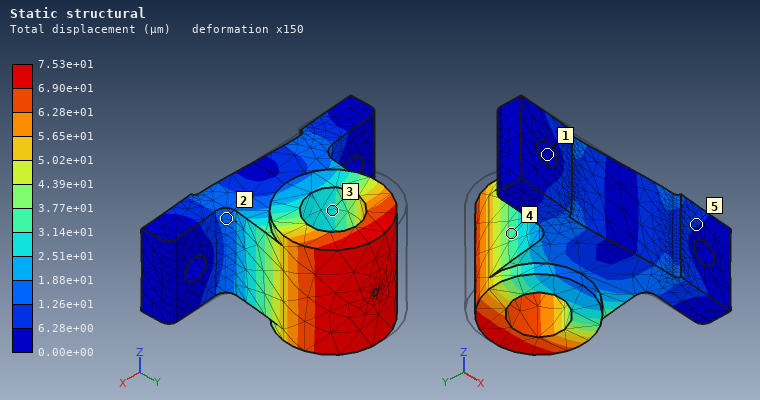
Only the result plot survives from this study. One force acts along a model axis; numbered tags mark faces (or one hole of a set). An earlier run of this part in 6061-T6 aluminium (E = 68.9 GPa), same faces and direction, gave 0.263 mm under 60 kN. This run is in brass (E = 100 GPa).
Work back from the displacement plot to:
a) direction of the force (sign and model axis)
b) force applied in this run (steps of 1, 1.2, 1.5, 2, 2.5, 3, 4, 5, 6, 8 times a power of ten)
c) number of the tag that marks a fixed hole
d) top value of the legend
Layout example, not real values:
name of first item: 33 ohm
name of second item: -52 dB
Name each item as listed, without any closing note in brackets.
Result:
direction of the force: +X
force applied in this run: 25 kN
number of the tag that marks a fixed hole: 1
top value of the legend: 7.53e+01 µm
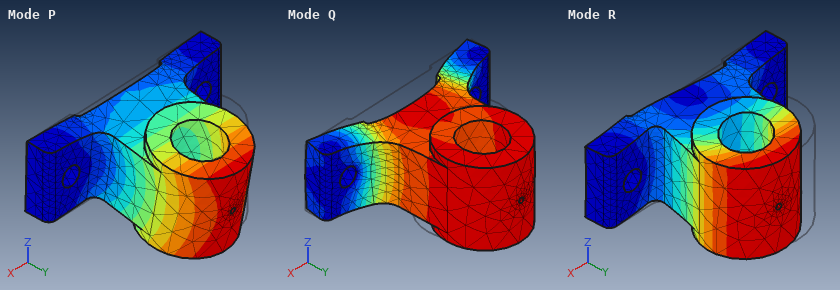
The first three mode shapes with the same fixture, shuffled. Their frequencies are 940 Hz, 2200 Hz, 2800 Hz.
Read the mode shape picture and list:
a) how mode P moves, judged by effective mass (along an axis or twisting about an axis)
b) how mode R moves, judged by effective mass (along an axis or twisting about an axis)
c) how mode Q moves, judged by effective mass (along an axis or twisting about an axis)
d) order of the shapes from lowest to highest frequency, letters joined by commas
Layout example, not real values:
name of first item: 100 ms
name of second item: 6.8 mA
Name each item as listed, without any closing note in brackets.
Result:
how mode P moves, judged by effective mass: along Z
how mode R moves, judged by effective mass: along X
how mode Q moves, judged by effective mass: along Y
order of the shapes from lowest to highest frequency, letters joined by commas: P, R, Q
